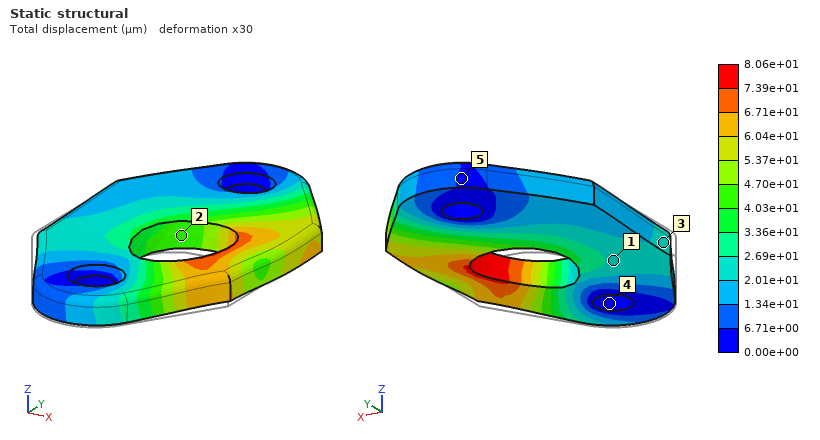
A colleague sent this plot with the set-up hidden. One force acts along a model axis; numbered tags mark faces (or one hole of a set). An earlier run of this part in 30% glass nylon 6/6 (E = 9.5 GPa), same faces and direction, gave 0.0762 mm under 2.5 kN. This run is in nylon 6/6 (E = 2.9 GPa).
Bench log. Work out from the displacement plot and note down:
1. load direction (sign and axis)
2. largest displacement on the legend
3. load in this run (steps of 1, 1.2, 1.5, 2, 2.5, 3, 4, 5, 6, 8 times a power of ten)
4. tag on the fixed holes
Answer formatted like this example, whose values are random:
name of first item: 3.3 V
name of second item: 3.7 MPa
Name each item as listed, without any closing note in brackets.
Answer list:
load direction: +Y
largest displacement on the legend: 8.06e+01 µm
load in this run: 800 N
tag on the fixed holes: 4
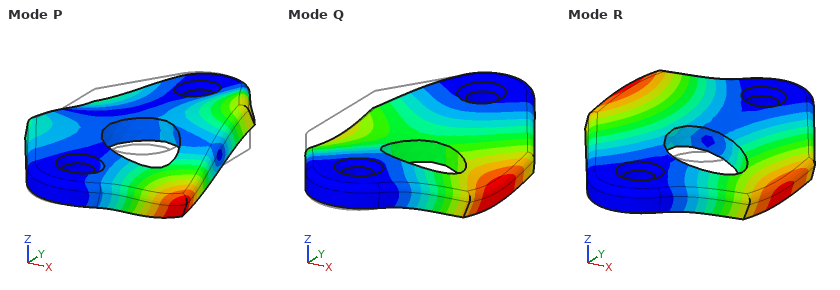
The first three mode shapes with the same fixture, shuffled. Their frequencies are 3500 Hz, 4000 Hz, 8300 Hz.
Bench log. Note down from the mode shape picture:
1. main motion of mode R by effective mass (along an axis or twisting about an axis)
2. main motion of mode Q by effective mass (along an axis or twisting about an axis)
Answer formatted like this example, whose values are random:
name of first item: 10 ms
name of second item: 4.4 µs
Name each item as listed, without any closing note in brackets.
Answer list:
main motion of mode R by effective mass: twisting about Y
main motion of mode Q by effective mass: along Z
